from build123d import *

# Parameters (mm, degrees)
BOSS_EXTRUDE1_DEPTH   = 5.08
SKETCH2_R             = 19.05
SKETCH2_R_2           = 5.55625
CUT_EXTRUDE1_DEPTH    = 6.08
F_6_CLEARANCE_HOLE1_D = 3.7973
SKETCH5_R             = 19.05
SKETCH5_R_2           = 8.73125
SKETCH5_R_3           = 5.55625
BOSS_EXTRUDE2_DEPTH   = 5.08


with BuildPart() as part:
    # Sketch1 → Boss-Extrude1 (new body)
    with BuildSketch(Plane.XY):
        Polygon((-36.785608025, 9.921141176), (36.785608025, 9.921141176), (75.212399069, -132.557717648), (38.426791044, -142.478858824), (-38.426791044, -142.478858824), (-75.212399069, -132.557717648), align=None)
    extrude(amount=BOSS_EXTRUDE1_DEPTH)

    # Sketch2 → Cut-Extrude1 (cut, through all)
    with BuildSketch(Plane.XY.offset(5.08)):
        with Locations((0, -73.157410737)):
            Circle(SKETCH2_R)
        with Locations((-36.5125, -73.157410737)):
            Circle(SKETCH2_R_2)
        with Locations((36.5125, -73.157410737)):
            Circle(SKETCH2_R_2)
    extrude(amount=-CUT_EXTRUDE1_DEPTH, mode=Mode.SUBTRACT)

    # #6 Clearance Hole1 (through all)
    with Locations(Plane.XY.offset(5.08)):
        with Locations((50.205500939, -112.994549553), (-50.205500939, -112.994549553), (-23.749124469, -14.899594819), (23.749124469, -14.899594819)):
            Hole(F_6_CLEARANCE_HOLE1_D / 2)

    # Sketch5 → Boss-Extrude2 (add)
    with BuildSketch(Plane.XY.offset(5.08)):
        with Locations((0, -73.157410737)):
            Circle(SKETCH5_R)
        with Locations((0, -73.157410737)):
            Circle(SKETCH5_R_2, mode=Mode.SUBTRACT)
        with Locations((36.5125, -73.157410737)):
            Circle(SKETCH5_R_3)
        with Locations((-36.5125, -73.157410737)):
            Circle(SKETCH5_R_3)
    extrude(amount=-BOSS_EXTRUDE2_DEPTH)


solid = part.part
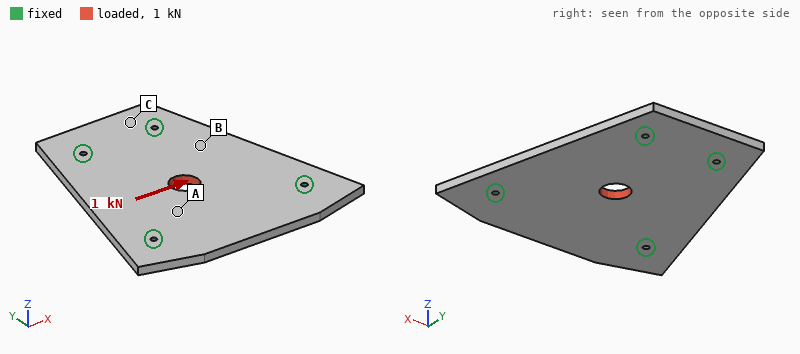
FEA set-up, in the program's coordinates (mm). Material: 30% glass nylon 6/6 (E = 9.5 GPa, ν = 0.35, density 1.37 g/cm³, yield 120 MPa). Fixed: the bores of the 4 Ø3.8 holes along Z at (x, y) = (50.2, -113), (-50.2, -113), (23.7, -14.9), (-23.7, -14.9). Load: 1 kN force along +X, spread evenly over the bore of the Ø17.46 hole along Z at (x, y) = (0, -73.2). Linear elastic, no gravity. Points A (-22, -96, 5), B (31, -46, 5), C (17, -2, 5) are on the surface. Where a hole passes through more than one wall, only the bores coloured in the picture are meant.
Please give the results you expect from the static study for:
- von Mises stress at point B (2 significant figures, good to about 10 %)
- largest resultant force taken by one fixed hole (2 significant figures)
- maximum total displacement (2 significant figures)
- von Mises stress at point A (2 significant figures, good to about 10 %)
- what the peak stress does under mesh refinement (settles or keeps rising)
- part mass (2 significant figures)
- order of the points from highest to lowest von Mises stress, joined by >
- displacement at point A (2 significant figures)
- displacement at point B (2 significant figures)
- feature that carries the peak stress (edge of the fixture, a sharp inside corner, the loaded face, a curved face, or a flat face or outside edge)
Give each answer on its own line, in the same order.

1.2 MPa
330 N
21 µm
2.2 MPa
keeps rising
120 g
A > B > C
10 µm
12 µm
edge of the fixture
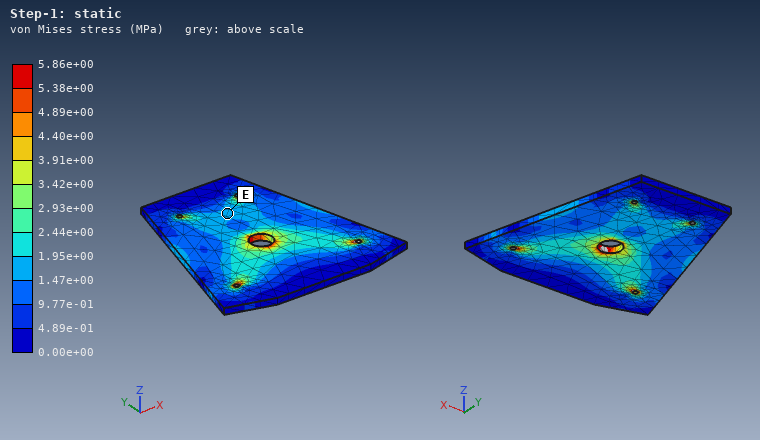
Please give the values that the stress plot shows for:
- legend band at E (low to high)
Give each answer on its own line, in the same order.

1.47e+00 to 1.95e+00 MPa
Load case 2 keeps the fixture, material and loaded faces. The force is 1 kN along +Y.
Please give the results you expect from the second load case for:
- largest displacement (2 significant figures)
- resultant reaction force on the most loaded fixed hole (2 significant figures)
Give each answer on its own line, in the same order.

18 µm
280 N
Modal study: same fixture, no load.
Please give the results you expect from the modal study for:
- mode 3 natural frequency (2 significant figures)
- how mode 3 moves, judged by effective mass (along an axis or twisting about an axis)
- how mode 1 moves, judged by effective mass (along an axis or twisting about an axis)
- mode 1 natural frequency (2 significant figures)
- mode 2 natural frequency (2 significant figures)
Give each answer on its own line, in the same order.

1400 Hz
twisting about Y
along Z
1000 Hz
1100 Hz
